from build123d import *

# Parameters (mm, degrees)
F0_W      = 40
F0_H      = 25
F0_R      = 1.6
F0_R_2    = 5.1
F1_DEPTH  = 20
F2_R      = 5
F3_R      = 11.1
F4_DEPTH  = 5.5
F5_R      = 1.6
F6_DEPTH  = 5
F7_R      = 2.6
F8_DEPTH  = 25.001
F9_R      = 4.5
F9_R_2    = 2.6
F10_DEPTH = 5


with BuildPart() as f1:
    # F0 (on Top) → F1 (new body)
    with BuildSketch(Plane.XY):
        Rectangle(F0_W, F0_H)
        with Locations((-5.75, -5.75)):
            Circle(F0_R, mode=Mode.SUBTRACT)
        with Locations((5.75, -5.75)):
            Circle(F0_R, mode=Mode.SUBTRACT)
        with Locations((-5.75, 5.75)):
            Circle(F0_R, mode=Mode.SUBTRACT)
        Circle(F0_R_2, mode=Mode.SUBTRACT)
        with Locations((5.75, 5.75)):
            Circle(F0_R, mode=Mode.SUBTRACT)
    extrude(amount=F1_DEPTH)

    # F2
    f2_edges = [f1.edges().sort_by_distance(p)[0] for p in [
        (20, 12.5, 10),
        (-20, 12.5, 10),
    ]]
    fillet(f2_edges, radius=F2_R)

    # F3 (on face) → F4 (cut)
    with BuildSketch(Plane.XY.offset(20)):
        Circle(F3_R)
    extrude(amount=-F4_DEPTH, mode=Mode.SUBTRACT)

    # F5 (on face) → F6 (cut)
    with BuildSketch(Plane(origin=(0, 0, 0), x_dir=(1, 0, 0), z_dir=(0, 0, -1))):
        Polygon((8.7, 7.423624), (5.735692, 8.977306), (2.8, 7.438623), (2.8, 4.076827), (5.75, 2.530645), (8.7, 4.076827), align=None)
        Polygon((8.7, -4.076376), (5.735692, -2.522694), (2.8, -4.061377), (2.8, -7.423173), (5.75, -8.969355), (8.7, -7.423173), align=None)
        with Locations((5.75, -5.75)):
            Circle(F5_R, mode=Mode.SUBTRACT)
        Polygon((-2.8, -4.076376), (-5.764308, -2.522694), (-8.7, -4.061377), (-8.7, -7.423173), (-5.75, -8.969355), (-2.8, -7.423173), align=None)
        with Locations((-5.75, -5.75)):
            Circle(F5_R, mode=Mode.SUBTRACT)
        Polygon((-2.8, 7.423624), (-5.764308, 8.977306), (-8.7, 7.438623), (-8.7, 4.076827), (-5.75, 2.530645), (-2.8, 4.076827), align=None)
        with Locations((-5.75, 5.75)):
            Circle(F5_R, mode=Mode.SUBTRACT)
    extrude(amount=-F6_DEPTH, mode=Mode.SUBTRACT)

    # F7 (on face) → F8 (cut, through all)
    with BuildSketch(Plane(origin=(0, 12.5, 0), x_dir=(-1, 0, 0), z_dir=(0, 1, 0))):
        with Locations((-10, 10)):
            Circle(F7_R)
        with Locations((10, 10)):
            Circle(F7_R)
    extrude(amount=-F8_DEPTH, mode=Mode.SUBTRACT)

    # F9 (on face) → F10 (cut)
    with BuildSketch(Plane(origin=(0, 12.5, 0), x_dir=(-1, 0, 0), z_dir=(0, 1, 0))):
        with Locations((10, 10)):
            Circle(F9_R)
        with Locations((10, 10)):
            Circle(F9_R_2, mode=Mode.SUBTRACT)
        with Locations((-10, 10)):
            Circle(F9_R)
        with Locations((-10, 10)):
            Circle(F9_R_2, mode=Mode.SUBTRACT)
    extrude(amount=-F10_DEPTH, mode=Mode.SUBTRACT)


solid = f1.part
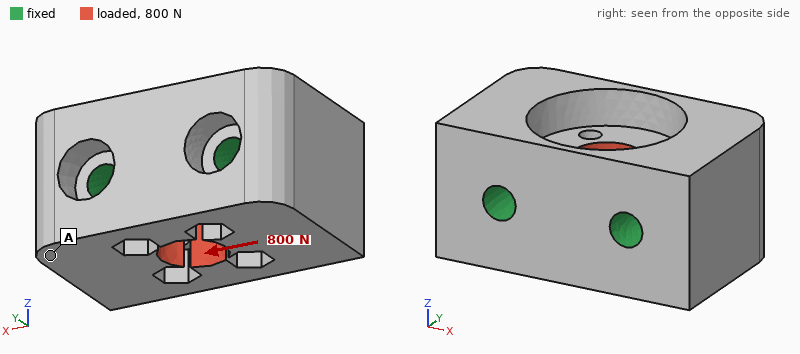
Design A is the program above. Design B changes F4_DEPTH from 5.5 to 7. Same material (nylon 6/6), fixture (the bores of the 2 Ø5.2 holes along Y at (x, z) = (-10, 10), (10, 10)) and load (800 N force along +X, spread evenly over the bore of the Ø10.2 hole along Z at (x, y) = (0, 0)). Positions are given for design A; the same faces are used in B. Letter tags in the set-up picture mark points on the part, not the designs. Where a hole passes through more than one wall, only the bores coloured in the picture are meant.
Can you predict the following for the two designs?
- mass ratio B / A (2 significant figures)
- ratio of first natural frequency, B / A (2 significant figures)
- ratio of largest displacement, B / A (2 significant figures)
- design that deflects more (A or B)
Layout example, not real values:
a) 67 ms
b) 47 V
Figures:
a) 0.97
b) 0.97
c) 1.1
d) B
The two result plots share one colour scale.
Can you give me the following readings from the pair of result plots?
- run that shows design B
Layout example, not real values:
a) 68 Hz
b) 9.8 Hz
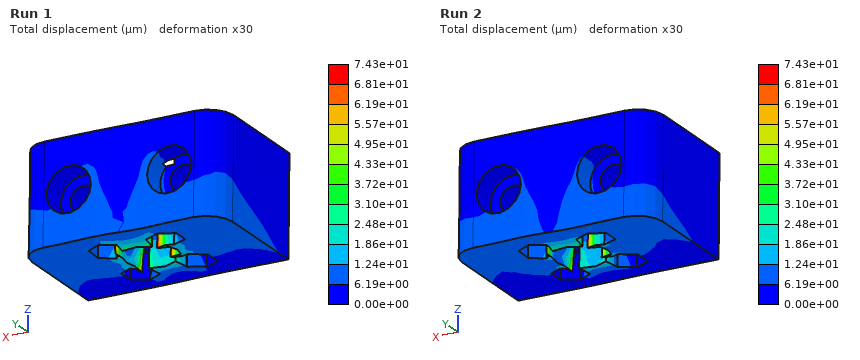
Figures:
a) Run 1
